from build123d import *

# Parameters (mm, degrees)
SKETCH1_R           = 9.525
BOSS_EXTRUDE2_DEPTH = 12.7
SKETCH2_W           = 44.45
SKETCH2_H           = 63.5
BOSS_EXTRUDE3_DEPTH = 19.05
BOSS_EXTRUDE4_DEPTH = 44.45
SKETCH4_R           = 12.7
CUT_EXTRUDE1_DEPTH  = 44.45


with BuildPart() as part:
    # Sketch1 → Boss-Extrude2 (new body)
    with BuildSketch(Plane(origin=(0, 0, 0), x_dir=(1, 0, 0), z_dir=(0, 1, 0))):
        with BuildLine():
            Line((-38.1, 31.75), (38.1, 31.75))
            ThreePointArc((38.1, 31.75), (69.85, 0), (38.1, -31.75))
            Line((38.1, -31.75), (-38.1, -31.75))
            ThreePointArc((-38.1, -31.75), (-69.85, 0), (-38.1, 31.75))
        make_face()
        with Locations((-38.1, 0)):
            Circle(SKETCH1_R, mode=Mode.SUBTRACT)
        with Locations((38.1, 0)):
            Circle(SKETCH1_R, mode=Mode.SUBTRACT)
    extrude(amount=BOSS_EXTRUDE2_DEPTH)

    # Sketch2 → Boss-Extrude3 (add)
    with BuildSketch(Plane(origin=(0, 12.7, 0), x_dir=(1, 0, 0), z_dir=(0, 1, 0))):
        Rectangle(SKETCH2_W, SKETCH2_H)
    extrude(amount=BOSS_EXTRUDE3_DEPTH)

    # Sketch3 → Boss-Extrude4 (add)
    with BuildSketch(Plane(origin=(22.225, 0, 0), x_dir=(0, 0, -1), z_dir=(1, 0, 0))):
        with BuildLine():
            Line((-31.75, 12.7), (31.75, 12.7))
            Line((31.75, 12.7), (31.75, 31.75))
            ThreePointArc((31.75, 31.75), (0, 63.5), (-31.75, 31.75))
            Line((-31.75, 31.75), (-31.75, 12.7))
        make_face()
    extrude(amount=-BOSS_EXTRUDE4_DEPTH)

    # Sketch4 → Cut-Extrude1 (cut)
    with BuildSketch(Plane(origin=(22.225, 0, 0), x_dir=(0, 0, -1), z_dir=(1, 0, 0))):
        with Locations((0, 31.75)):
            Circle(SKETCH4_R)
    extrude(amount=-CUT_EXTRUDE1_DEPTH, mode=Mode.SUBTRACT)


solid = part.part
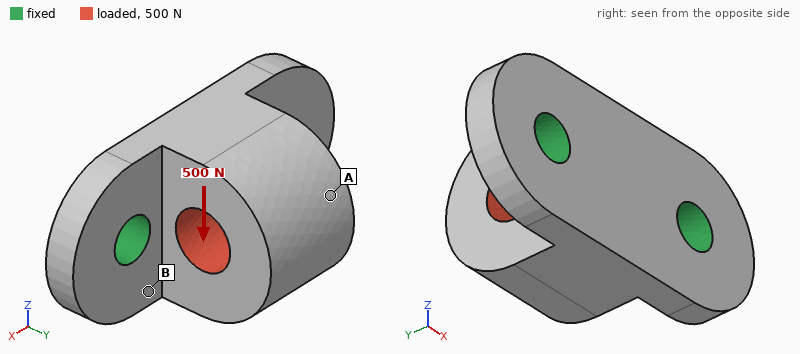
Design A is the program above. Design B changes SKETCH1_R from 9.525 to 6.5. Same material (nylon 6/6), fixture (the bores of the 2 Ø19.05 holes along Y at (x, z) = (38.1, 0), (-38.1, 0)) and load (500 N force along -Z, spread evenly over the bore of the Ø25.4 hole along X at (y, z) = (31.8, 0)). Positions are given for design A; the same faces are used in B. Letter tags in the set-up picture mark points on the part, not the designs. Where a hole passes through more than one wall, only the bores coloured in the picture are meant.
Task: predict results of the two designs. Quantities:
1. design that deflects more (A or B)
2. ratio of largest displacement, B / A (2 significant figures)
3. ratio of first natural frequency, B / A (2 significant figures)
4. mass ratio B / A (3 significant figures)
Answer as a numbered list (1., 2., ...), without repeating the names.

1. B
2. 1.4
3. 0.84
4. 1.02
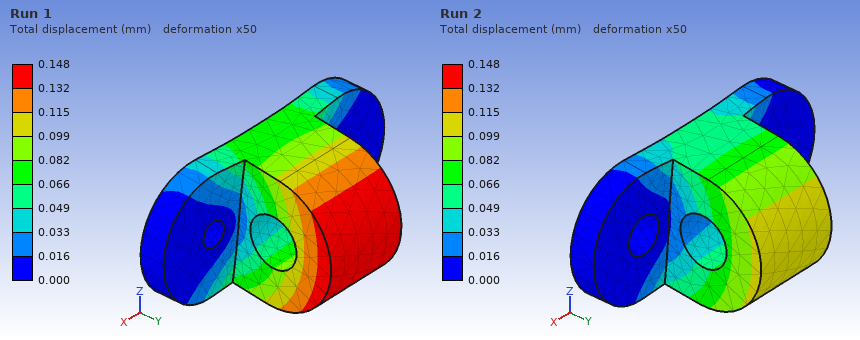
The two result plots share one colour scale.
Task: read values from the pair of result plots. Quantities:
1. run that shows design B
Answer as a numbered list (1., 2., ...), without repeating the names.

1. Run 1
